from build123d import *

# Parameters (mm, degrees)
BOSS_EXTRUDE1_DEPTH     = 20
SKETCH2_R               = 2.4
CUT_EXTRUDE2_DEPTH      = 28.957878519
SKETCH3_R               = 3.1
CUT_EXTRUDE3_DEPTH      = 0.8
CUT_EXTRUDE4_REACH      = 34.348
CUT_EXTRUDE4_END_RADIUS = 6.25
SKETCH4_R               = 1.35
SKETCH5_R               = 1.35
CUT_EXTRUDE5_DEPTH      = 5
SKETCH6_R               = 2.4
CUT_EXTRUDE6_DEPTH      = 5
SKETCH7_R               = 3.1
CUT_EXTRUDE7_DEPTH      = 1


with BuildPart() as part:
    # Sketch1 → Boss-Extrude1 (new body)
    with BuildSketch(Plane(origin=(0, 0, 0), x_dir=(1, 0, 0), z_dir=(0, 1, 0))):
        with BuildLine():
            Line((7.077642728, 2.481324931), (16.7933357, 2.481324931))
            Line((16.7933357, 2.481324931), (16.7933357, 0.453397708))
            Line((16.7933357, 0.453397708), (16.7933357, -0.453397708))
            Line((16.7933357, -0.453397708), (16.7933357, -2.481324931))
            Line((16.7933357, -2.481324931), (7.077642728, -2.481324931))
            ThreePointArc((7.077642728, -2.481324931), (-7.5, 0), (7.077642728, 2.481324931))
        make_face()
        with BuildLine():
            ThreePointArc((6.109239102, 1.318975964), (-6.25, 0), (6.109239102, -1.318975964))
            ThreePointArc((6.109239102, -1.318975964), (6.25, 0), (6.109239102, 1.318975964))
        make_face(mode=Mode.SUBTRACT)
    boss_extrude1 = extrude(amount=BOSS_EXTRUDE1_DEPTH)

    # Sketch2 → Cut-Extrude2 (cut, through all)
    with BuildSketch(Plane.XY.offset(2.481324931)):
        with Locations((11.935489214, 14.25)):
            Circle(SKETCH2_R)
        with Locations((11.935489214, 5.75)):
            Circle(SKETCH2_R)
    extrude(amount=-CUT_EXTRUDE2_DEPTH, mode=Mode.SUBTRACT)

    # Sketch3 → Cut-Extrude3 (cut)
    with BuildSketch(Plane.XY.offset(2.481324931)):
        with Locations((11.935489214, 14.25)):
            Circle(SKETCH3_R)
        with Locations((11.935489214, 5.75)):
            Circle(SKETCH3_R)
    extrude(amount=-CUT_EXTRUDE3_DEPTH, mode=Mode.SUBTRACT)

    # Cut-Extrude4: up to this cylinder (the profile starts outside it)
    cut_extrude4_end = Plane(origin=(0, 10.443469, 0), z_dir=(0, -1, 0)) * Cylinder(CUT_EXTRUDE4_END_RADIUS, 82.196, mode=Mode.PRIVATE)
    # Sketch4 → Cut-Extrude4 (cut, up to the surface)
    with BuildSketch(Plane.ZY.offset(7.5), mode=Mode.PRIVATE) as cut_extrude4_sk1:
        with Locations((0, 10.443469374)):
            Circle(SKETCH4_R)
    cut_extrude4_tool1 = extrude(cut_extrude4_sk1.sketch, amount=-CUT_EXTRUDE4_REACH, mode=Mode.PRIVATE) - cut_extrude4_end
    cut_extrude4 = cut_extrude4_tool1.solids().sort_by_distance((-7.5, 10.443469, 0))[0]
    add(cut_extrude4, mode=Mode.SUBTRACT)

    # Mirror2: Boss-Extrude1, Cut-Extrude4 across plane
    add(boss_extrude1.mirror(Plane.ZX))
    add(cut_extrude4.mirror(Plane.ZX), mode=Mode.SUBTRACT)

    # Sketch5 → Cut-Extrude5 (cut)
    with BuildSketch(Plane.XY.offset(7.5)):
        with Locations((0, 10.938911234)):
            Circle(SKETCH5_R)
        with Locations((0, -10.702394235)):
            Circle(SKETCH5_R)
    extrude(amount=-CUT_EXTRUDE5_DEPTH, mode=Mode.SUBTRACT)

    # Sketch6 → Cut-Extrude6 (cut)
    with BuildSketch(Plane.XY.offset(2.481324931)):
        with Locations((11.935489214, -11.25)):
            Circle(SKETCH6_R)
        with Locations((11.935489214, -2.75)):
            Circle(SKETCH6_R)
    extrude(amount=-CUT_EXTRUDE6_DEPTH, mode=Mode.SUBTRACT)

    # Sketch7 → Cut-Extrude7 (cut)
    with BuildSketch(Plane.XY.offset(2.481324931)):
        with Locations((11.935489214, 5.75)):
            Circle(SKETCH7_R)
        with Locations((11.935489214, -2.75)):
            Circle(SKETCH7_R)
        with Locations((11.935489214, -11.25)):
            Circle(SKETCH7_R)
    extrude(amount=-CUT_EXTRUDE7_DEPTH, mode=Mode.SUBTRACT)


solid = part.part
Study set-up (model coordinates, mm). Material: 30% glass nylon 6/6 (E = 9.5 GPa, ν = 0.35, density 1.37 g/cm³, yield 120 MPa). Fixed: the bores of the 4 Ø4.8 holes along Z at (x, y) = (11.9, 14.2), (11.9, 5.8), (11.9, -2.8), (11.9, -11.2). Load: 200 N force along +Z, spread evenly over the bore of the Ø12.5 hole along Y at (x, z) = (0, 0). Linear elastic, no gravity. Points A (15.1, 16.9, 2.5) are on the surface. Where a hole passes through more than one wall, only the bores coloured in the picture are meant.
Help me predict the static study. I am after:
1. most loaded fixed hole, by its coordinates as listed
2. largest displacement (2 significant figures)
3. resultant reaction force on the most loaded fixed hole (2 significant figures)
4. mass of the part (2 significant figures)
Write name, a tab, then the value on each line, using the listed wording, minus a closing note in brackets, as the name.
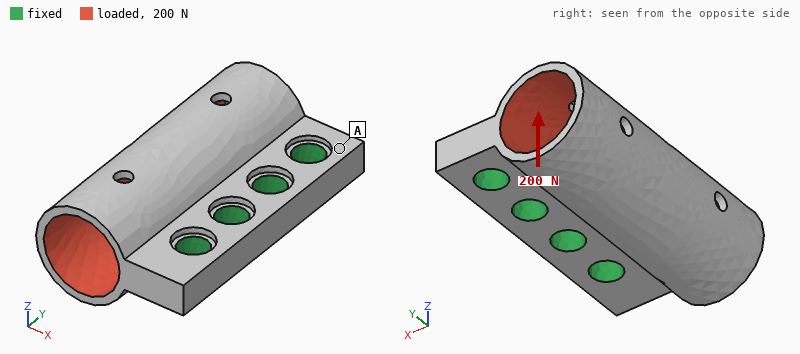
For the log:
most loaded fixed hole, by its coordinates as listed	(11.9, -11.2)
largest displacement	0.36 mm
resultant reaction force on the most loaded fixed hole	64 N
mass of the part	4.9 g
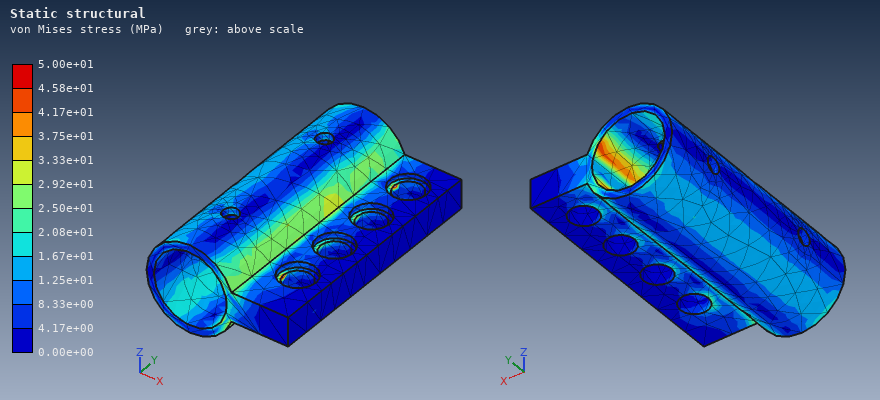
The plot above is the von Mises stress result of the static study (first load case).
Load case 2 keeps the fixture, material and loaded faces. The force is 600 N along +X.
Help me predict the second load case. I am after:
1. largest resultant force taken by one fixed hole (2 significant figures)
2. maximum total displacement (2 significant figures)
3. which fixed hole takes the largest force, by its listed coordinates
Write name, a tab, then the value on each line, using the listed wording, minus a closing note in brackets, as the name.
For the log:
largest resultant force taken by one fixed hole	210 N
maximum total displacement	0.14 mm
which fixed hole takes the largest force, by its listed coordinates	(11.9, -11.2)
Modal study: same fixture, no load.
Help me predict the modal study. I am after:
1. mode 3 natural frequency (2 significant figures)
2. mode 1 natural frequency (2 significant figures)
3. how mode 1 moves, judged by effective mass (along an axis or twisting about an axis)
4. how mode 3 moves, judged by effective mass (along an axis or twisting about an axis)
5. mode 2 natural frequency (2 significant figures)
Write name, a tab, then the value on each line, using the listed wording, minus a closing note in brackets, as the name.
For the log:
mode 3 natural frequency	6700 Hz
mode 1 natural frequency	2400 Hz
how mode 1 moves, judged by effective mass	along Z
how mode 3 moves, judged by effective mass	along X
mode 2 natural frequency	6200 Hz
